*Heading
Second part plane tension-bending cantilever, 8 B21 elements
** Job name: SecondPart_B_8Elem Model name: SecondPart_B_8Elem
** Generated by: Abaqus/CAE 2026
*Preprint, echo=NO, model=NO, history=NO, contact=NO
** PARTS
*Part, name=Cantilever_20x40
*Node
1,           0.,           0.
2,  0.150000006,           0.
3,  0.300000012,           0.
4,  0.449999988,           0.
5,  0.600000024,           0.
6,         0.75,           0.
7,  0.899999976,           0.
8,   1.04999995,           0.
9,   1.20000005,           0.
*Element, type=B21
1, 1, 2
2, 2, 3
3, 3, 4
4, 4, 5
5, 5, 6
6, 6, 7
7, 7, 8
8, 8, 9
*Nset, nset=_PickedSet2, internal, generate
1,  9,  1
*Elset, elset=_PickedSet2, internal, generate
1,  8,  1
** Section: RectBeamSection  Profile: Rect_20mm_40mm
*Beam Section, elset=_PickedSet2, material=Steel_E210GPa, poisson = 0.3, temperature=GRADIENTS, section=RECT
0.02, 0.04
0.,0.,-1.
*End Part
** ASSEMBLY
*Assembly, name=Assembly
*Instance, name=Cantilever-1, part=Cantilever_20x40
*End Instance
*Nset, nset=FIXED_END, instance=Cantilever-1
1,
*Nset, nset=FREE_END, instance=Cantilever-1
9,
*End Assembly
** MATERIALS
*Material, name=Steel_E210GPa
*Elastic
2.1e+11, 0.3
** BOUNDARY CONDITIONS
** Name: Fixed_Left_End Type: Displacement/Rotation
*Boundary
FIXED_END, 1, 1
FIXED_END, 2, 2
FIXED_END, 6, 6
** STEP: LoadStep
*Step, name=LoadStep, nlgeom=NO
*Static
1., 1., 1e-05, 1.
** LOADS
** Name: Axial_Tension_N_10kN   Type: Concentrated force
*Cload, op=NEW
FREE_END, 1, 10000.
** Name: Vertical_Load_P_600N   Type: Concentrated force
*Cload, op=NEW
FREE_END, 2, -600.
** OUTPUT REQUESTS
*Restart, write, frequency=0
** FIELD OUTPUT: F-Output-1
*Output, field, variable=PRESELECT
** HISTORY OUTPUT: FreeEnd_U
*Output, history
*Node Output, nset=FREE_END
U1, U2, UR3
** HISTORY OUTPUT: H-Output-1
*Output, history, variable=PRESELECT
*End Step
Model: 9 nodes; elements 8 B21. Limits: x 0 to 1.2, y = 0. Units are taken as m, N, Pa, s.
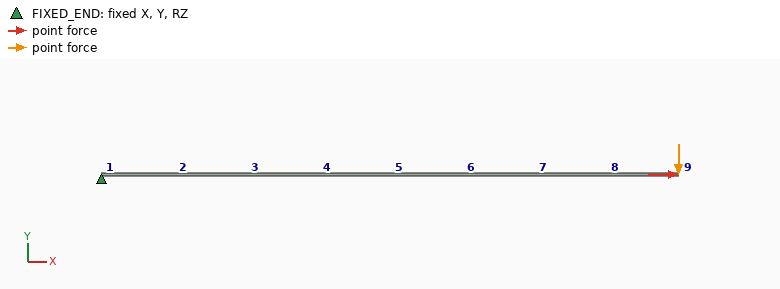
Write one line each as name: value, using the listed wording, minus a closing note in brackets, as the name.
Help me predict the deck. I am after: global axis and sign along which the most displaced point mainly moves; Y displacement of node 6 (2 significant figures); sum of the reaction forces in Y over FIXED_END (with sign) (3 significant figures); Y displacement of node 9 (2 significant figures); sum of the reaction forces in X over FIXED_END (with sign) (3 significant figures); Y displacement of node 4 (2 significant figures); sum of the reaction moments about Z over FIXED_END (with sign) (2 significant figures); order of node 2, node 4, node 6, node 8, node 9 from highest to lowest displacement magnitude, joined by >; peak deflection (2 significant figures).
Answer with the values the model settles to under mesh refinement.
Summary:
global axis and sign along which the most displaced point mainly moves: -Y
Y displacement of node 6: -0.0072 m
sum of the reaction forces in Y over FIXED_END (with sign): 600 N
Y displacement of node 9: -0.015 m
sum of the reaction forces in X over FIXED_END (with sign): -10000 N
Y displacement of node 4: -0.0029 m
sum of the reaction moments about Z over FIXED_END (with sign): 720 N·m
order of node 2, node 4, node 6, node 8, node 9 from highest to lowest displacement magnitude, joined by >: node 9 > node 8 > node 6 > node 4 > node 2
peak deflection: 0.015 m
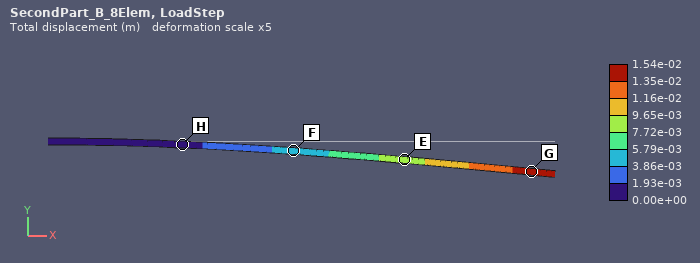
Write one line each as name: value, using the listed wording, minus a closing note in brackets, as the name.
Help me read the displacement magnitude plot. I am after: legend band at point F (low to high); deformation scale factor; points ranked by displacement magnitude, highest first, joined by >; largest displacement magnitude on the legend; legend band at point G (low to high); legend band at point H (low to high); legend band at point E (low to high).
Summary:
legend band at point F: 3.86e-03 to 5.79e-03 m
deformation scale factor: 5
points ranked by displacement magnitude, highest first, joined by >: G > E > F > H
largest displacement magnitude on the legend: 1.54e-02 m
legend band at point G: 1.35e-02 to 1.54e-02 m
legend band at point H: 0.00e+00 to 1.93e-03 m
legend band at point E: 7.72e-03 to 9.65e-03 m
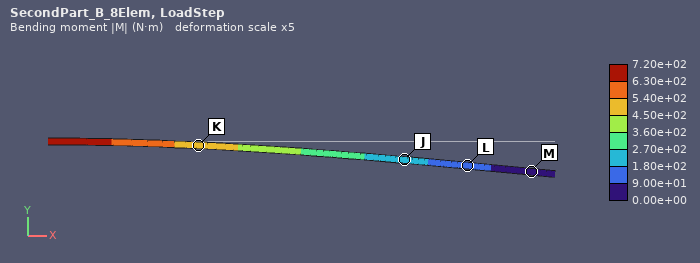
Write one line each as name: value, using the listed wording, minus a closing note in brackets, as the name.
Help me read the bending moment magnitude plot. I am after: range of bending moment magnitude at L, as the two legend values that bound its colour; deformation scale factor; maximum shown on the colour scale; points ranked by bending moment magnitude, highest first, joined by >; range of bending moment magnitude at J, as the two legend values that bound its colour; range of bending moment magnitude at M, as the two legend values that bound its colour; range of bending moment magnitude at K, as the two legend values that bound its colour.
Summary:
range of bending moment magnitude at L, as the two legend values that bound its colour: 9.00e+01 to 1.80e+02 N·m
deformation scale factor: 5
maximum shown on the colour scale: 7.20e+02 N·m
points ranked by bending moment magnitude, highest first, joined by >: K > J > L > M
range of bending moment magnitude at J, as the two legend values that bound its colour: 1.80e+02 to 2.70e+02 N·m
range of bending moment magnitude at M, as the two legend values that bound its colour: 0.00e+00 to 9.00e+01 N·m
range of bending moment magnitude at K, as the two legend values that bound its colour: 4.50e+02 to 5.40e+02 N·m
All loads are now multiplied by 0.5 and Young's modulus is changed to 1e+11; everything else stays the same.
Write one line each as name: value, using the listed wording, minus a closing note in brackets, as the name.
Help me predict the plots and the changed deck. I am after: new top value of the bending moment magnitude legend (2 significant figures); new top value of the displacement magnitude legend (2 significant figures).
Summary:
new top value of the bending moment magnitude legend: 360 N·m
new top value of the displacement magnitude legend: 0.016 m
